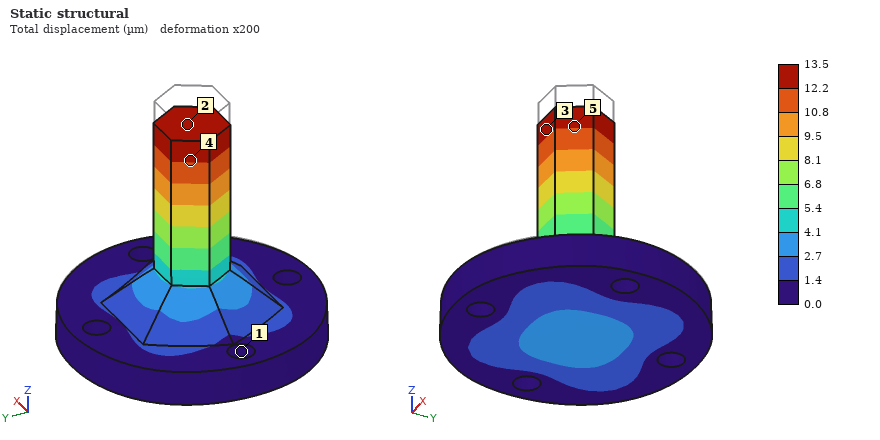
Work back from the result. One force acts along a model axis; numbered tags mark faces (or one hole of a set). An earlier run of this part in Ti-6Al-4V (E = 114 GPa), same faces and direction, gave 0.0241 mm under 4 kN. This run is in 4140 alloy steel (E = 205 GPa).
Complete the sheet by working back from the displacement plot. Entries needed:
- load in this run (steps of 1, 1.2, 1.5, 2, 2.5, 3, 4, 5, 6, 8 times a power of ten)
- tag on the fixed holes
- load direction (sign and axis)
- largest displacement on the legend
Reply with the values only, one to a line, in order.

4 kN
1
-Z
13.5 µm
